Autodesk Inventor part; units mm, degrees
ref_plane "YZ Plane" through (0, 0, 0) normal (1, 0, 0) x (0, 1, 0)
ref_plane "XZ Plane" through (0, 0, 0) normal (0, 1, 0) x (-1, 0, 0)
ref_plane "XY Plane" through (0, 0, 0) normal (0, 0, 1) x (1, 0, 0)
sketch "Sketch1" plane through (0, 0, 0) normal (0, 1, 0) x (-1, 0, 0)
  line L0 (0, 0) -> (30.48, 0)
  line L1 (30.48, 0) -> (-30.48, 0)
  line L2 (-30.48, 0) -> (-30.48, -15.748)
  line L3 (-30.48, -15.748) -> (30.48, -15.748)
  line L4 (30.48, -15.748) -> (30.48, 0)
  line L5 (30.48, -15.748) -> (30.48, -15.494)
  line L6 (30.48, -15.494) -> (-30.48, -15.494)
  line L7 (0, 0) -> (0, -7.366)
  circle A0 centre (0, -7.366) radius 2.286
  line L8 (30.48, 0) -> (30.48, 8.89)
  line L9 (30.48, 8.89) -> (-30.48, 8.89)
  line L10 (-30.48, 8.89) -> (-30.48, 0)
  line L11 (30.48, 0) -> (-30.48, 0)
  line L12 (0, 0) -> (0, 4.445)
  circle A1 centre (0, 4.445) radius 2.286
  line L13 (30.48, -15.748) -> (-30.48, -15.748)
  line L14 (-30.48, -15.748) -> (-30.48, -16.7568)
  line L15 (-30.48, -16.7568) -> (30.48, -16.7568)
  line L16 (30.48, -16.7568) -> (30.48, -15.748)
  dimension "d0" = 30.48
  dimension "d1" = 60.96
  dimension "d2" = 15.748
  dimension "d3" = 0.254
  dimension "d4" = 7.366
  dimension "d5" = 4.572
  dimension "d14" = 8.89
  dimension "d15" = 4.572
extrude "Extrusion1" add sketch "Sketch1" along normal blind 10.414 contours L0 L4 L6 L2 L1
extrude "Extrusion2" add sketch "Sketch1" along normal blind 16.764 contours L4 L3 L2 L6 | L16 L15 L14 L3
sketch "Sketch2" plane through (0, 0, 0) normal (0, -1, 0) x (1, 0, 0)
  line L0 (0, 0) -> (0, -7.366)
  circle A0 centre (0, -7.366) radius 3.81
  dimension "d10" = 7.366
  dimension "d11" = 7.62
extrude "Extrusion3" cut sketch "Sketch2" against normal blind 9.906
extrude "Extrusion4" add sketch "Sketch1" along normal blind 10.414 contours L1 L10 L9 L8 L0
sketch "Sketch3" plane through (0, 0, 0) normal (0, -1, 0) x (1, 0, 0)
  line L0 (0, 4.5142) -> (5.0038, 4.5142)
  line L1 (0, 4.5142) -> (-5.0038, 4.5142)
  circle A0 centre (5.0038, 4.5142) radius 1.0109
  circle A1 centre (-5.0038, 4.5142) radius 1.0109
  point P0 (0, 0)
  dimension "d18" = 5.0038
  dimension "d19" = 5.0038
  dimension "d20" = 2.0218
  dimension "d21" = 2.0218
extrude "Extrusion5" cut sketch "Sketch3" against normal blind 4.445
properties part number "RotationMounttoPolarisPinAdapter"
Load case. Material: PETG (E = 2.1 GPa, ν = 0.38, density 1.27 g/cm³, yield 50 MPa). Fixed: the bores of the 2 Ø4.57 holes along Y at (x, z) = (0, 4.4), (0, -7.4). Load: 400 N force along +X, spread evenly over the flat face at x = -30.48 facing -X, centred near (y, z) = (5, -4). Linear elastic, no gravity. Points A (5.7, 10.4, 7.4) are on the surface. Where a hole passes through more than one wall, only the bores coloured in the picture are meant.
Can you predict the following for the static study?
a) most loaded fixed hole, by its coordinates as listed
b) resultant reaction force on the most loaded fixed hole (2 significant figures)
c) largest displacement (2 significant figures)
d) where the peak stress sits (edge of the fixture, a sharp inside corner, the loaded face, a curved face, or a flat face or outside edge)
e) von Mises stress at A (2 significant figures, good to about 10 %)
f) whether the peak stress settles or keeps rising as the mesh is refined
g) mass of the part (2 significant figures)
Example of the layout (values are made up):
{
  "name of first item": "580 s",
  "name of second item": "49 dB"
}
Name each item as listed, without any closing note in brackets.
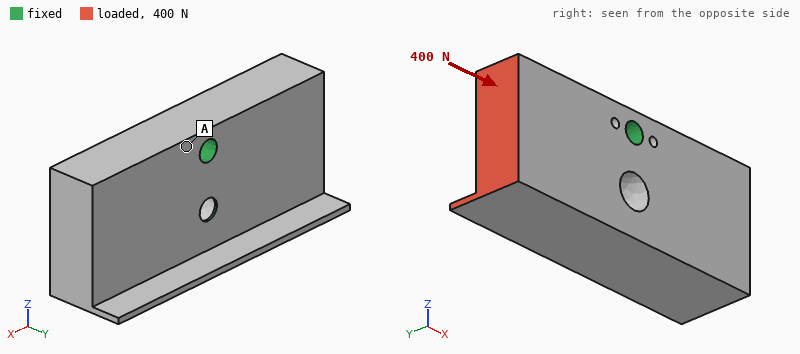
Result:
{
  "most loaded fixed hole, by its coordinates as listed": "(0, 4.4)",
  "resultant reaction force on the most loaded fixed hole": "230 N",
  "largest displacement": "0.15 mm",
  "where the peak stress sits": "edge of the fixture",
  "von Mises stress at A": "2.3 MPa",
  "whether the peak stress settles or keeps rising as the mesh is refined": "keeps rising",
  "mass of the part": "20 g"
}
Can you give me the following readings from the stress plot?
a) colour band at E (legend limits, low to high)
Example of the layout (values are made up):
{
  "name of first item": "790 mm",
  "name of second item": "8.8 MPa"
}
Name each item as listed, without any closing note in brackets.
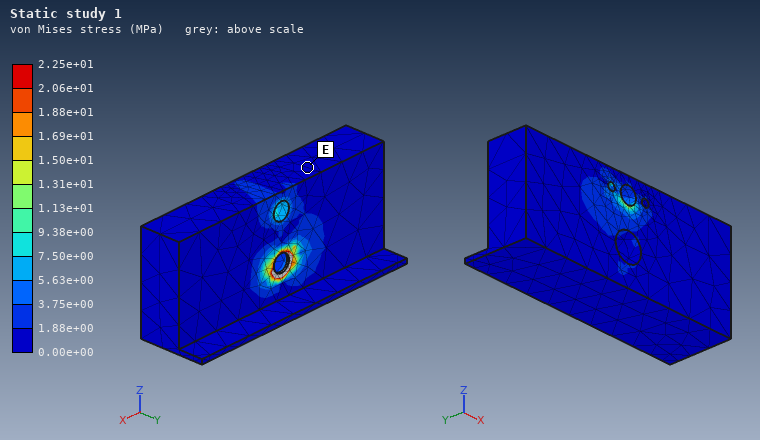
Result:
{
  "colour band at E": "0.00e+00 to 1.88e+00 MPa"
}
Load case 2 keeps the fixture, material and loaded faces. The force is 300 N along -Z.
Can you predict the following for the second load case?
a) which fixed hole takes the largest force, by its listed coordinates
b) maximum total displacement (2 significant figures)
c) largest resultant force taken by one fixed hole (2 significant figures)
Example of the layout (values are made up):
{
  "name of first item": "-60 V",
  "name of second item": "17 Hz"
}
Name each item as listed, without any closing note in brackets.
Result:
{
  "which fixed hole takes the largest force, by its listed coordinates": "(0, 4.4)",
  "maximum total displacement": "0.66 mm",
  "largest resultant force taken by one fixed hole": "490 N"
}
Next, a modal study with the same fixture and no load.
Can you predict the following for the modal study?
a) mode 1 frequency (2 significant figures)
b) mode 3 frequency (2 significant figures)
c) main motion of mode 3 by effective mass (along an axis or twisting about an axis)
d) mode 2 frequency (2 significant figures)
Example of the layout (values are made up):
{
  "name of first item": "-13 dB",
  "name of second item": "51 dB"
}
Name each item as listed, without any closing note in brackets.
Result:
{
  "mode 1 frequency": "1300 Hz",
  "mode 3 frequency": "2000 Hz",
  "main motion of mode 3 by effective mass": "along Y",
  "mode 2 frequency": "1900 Hz"
}
